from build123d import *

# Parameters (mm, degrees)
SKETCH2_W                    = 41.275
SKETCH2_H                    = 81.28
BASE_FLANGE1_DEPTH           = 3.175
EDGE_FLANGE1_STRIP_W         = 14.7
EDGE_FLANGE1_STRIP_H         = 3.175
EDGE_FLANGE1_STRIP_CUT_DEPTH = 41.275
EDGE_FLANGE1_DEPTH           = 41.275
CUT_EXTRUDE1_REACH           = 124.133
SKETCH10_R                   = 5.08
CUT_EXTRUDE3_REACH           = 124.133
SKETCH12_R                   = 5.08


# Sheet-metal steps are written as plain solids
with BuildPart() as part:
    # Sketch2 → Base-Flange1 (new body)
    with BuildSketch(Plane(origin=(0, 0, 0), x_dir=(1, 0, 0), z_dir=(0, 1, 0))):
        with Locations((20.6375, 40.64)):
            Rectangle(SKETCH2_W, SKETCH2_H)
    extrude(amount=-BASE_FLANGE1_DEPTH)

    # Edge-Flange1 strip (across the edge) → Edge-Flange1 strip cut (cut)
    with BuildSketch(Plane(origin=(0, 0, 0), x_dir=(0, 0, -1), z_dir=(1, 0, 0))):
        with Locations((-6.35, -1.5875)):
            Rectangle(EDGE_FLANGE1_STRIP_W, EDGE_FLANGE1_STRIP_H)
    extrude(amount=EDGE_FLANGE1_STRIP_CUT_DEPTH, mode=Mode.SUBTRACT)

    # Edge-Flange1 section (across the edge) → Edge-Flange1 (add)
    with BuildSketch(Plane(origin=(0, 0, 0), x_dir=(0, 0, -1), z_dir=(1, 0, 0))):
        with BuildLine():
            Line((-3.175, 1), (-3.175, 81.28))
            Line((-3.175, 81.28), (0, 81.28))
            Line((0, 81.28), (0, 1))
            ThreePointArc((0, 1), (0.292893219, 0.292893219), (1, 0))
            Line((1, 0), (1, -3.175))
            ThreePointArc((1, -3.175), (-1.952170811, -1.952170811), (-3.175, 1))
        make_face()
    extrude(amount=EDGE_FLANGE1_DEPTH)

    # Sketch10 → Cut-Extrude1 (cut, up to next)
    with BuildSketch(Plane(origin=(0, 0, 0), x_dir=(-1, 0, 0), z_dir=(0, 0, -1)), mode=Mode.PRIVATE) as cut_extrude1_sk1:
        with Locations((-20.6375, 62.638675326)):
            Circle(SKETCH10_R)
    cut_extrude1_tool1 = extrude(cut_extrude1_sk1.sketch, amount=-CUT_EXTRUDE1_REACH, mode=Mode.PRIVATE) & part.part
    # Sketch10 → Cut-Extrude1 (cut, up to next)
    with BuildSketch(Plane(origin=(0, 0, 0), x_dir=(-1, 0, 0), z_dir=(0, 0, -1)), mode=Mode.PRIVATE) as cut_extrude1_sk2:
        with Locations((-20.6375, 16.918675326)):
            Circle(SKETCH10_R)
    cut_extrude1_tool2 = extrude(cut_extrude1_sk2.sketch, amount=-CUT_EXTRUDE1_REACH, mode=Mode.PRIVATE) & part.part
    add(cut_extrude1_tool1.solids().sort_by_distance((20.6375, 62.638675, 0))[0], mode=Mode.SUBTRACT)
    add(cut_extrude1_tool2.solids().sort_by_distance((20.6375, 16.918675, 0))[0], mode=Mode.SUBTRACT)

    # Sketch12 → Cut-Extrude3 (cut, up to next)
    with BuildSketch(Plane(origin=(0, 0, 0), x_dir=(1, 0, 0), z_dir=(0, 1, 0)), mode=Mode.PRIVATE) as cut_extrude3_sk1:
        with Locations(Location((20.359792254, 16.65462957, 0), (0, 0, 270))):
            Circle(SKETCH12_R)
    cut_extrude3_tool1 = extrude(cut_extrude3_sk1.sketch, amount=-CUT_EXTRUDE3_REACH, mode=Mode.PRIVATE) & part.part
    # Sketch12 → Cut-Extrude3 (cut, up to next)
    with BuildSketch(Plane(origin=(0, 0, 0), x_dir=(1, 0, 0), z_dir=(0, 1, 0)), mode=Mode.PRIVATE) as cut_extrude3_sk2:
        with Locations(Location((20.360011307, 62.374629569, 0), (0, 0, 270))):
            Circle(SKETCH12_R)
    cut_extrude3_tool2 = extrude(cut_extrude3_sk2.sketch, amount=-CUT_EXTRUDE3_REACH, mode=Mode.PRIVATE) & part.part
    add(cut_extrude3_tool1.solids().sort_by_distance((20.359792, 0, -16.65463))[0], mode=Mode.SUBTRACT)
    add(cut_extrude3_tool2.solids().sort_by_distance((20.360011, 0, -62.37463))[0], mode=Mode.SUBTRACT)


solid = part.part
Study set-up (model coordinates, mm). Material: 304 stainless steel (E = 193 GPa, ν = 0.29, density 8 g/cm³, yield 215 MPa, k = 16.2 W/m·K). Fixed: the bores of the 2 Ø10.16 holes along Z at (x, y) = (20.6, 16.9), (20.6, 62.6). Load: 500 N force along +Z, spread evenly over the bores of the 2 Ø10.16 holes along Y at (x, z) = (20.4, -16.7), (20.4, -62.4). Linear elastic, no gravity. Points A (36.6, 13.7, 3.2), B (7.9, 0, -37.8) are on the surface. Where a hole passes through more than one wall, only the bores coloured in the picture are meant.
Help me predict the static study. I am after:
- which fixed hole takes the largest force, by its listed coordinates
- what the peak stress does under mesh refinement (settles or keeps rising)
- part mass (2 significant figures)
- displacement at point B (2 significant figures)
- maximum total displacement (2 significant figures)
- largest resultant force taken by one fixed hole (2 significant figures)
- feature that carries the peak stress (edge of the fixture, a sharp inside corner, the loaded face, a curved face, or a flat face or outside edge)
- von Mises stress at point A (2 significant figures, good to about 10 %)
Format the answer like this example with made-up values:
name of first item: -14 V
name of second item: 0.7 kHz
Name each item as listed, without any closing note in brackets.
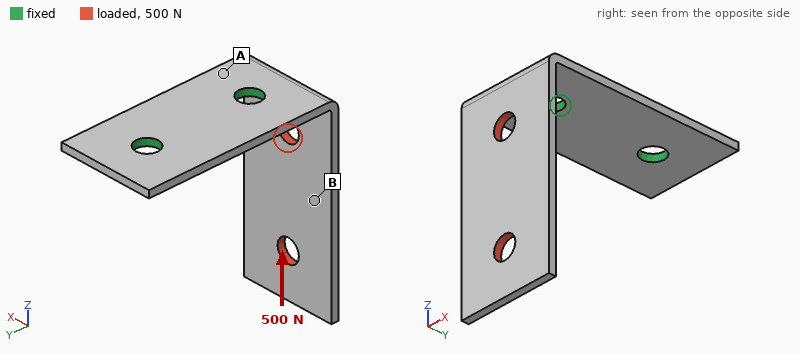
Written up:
which fixed hole takes the largest force, by its listed coordinates: (20.6, 16.9)
what the peak stress does under mesh refinement: keeps rising
part mass: 160 g
displacement at point B: 0.12 mm
maximum total displacement: 0.25 mm
largest resultant force taken by one fixed hole: 520 N
feature that carries the peak stress: edge of the fixture
von Mises stress at point A: 43 MPa
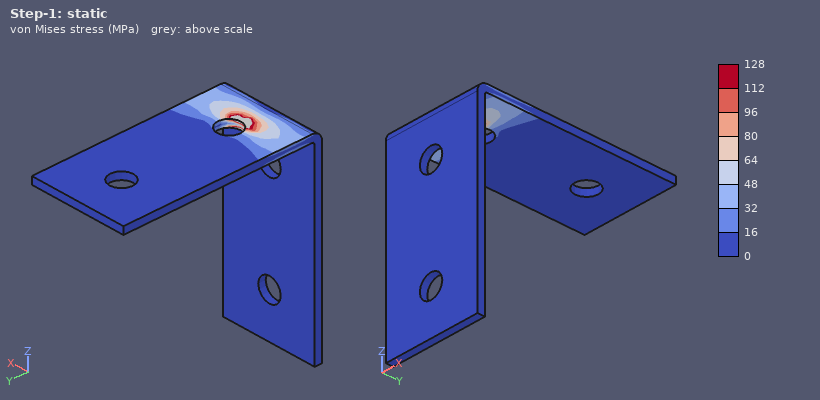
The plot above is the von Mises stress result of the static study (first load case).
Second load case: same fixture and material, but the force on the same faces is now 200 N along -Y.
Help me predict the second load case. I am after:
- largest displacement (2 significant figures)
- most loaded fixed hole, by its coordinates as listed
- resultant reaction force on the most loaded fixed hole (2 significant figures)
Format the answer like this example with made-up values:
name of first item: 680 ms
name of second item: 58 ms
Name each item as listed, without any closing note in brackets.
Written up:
largest displacement: 1.2 mm
most loaded fixed hole, by its coordinates as listed: (20.6, 16.9)
resultant reaction force on the most loaded fixed hole: 190 N
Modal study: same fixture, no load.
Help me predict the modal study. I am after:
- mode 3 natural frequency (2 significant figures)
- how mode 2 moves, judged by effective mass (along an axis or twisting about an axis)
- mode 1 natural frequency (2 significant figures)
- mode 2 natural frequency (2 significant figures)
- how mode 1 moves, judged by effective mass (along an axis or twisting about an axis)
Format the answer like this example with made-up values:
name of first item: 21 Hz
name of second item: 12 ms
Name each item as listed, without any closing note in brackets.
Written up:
mode 3 natural frequency: 1500 Hz
how mode 2 moves, judged by effective mass: along X
mode 1 natural frequency: 280 Hz
mode 2 natural frequency: 600 Hz
how mode 1 moves, judged by effective mass: along Y
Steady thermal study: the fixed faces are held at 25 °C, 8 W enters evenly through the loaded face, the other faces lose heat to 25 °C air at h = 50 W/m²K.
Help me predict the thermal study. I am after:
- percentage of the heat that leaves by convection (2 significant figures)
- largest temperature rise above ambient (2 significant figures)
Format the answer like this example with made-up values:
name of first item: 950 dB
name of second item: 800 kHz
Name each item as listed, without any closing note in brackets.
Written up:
percentage of the heat that leaves by convection: 89 %
largest temperature rise above ambient: 33 K
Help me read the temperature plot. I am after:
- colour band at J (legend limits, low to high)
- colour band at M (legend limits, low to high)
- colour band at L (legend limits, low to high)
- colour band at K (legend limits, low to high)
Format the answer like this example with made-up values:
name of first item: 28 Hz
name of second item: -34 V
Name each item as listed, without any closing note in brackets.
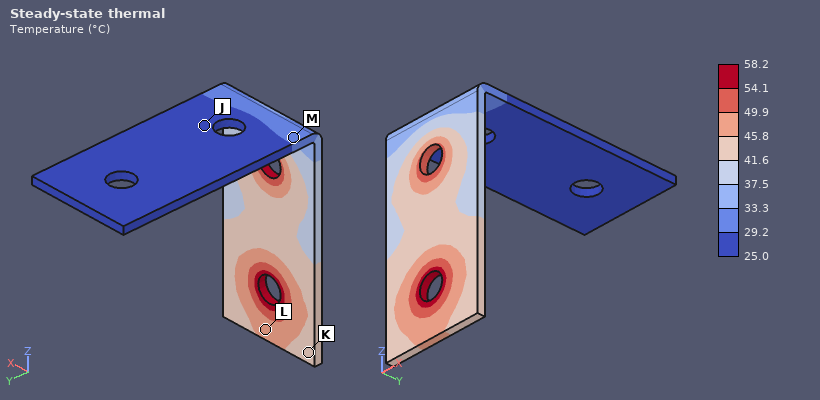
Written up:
colour band at J: 25.0 to 29.2 °C
colour band at M: 29.2 to 33.3 °C
colour band at L: 45.8 to 49.9 °C
colour band at K: 41.6 to 45.8 °C
